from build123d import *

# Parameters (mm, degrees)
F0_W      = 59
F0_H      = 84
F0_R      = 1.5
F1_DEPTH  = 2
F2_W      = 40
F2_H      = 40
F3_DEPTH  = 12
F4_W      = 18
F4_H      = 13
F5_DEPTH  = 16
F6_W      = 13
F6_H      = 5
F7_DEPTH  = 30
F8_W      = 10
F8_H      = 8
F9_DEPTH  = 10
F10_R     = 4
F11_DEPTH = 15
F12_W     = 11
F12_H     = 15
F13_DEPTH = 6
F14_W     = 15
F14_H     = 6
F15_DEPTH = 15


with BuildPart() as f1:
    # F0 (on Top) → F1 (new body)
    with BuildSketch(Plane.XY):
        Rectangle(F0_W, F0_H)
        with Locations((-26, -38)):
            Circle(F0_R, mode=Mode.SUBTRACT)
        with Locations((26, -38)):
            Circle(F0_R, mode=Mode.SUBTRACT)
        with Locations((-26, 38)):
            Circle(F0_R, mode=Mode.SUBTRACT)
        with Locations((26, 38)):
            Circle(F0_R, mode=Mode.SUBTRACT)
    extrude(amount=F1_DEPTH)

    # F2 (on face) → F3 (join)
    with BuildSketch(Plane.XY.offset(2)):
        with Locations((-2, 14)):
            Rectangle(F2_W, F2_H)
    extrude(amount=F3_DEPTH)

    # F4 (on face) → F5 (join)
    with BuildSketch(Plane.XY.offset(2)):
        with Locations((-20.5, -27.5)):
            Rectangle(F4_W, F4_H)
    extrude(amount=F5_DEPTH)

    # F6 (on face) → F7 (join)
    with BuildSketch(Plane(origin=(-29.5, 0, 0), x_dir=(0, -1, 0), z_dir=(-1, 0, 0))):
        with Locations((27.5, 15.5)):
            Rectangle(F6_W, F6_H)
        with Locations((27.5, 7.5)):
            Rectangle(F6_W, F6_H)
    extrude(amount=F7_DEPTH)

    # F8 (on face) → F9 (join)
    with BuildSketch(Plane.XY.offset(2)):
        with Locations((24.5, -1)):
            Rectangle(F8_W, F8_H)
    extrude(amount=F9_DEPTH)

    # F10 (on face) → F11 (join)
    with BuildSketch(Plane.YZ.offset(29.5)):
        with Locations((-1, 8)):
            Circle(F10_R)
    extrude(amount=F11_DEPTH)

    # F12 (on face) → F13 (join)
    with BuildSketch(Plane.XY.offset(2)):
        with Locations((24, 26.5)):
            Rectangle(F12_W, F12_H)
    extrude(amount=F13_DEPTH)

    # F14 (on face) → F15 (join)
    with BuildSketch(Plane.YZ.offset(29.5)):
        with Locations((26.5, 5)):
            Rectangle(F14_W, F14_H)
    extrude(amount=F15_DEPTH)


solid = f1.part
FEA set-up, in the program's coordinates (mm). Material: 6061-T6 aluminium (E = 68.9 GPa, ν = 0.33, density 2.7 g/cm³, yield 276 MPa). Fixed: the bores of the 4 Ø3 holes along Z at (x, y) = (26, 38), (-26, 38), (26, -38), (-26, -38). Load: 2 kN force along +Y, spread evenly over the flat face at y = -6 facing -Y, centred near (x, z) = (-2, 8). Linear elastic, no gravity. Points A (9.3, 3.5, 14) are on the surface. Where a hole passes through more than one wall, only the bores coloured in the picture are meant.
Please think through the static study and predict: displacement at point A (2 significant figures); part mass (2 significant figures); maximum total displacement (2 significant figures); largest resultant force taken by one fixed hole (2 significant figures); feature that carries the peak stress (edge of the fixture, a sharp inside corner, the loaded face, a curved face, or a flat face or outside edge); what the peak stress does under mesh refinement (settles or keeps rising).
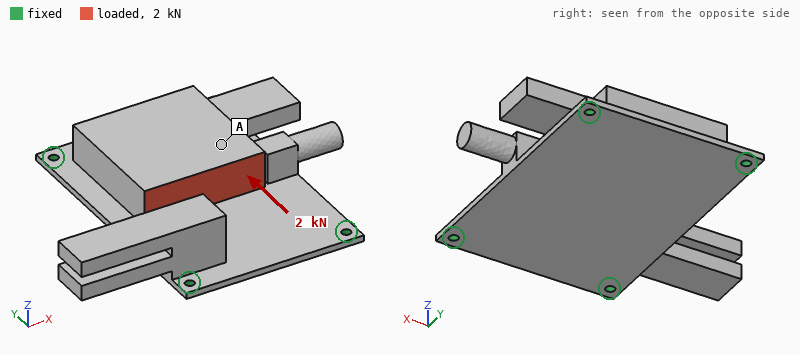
0.17 mm
110 g
0.22 mm
650 N
edge of the fixture
keeps rising
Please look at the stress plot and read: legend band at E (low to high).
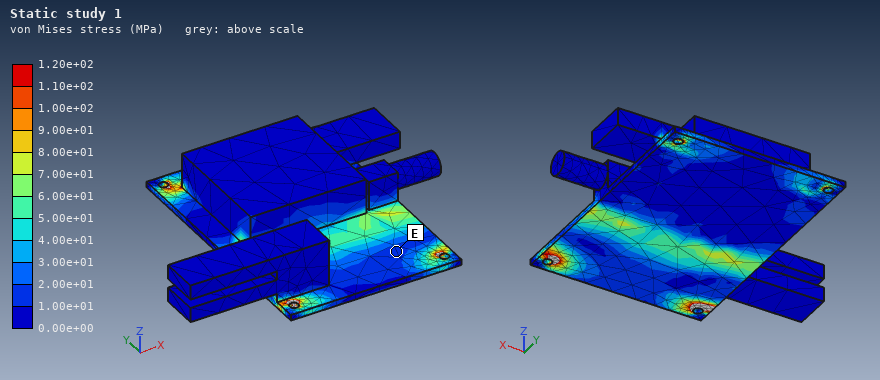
1.00e+01 to 2.00e+01 MPa
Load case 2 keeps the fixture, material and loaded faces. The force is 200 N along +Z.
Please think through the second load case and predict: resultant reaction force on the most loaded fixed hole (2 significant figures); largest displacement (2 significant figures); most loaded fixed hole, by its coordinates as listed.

68 N
0.14 mm
(-26, -38)
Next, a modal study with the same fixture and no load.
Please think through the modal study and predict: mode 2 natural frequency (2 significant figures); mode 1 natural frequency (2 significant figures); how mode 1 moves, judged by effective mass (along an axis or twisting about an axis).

1400 Hz
970 Hz
along Z
